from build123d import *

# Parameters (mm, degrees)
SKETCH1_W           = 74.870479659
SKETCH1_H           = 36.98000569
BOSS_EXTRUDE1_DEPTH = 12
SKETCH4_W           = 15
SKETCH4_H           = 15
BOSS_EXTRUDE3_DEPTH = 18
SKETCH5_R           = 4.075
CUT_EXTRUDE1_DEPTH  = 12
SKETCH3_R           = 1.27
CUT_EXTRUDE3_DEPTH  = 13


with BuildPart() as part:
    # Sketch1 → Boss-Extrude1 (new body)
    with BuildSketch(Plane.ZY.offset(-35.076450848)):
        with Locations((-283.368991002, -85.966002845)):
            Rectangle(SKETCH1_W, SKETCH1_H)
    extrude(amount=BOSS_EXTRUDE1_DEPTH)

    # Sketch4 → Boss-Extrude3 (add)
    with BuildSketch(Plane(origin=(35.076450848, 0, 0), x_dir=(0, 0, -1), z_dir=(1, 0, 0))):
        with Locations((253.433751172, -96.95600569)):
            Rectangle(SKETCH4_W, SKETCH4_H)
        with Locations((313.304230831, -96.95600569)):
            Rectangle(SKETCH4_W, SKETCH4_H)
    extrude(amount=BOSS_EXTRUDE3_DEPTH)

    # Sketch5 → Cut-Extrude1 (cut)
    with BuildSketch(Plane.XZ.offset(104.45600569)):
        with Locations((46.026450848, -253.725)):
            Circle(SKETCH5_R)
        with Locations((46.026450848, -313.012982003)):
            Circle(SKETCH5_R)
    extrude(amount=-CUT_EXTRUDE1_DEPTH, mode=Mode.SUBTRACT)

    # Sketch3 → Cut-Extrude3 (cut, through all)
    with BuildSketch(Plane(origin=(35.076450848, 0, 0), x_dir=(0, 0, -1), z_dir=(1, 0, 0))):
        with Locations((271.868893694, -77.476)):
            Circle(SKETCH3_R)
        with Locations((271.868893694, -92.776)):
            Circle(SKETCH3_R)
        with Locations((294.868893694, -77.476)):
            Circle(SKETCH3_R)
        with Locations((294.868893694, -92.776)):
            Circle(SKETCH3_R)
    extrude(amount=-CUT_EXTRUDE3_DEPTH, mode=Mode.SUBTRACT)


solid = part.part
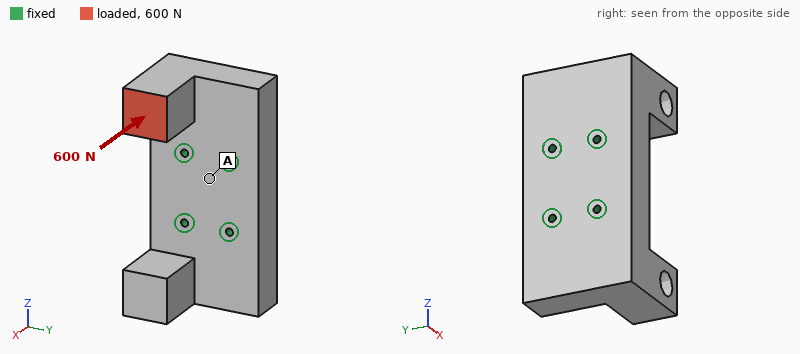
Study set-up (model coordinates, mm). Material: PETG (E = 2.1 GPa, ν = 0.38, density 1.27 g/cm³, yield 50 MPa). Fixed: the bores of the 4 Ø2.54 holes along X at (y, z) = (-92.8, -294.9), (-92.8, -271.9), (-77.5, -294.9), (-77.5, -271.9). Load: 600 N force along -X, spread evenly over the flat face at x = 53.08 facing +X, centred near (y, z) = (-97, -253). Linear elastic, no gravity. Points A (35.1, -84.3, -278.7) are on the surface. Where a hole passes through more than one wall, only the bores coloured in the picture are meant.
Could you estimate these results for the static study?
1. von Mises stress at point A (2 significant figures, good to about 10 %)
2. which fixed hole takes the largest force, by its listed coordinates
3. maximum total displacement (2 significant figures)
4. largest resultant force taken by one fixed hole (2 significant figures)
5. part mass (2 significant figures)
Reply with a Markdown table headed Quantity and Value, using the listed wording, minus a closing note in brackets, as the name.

| Quantity | Value |
|---|---|
| von Mises stress at point A | 3.2 MPa |
| which fixed hole takes the largest force, by its listed coordinates | (-92.8, -271.9) |
| maximum total displacement | 0.60 mm |
| largest resultant force taken by one fixed hole | 660 N |
| part mass | 51 g |
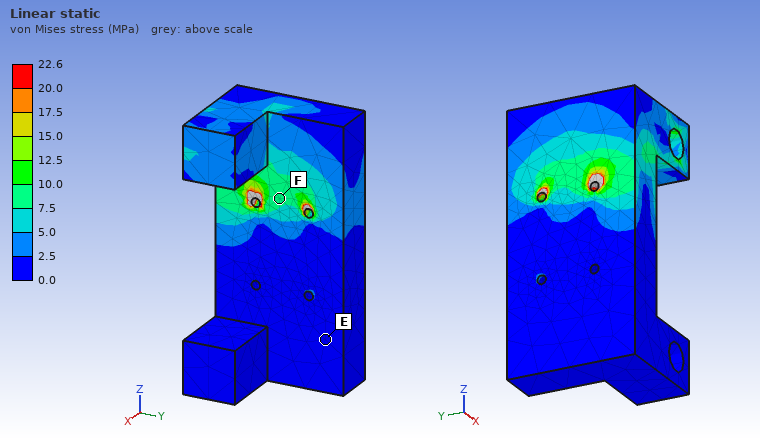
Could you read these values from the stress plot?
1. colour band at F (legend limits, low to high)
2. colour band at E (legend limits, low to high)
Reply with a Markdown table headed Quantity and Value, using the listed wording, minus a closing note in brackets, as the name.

| Quantity | Value |
|---|---|
| colour band at F | 7.5 to 10.0 MPa |
| colour band at E | 0.0 to 2.5 MPa |
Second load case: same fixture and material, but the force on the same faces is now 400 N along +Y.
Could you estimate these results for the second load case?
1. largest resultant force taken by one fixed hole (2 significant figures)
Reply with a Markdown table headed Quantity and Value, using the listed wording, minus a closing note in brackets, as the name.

| Quantity | Value |
|---|---|
| largest resultant force taken by one fixed hole | 500 N |
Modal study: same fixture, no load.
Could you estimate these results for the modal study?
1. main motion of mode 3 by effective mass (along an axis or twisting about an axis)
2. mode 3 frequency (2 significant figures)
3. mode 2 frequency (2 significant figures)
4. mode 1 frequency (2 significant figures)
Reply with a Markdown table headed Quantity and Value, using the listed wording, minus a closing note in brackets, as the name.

| Quantity | Value |
|---|---|
| main motion of mode 3 by effective mass | twisting about X |
| mode 3 frequency | 2600 Hz |
| mode 2 frequency | 1900 Hz |
| mode 1 frequency | 1900 Hz |
